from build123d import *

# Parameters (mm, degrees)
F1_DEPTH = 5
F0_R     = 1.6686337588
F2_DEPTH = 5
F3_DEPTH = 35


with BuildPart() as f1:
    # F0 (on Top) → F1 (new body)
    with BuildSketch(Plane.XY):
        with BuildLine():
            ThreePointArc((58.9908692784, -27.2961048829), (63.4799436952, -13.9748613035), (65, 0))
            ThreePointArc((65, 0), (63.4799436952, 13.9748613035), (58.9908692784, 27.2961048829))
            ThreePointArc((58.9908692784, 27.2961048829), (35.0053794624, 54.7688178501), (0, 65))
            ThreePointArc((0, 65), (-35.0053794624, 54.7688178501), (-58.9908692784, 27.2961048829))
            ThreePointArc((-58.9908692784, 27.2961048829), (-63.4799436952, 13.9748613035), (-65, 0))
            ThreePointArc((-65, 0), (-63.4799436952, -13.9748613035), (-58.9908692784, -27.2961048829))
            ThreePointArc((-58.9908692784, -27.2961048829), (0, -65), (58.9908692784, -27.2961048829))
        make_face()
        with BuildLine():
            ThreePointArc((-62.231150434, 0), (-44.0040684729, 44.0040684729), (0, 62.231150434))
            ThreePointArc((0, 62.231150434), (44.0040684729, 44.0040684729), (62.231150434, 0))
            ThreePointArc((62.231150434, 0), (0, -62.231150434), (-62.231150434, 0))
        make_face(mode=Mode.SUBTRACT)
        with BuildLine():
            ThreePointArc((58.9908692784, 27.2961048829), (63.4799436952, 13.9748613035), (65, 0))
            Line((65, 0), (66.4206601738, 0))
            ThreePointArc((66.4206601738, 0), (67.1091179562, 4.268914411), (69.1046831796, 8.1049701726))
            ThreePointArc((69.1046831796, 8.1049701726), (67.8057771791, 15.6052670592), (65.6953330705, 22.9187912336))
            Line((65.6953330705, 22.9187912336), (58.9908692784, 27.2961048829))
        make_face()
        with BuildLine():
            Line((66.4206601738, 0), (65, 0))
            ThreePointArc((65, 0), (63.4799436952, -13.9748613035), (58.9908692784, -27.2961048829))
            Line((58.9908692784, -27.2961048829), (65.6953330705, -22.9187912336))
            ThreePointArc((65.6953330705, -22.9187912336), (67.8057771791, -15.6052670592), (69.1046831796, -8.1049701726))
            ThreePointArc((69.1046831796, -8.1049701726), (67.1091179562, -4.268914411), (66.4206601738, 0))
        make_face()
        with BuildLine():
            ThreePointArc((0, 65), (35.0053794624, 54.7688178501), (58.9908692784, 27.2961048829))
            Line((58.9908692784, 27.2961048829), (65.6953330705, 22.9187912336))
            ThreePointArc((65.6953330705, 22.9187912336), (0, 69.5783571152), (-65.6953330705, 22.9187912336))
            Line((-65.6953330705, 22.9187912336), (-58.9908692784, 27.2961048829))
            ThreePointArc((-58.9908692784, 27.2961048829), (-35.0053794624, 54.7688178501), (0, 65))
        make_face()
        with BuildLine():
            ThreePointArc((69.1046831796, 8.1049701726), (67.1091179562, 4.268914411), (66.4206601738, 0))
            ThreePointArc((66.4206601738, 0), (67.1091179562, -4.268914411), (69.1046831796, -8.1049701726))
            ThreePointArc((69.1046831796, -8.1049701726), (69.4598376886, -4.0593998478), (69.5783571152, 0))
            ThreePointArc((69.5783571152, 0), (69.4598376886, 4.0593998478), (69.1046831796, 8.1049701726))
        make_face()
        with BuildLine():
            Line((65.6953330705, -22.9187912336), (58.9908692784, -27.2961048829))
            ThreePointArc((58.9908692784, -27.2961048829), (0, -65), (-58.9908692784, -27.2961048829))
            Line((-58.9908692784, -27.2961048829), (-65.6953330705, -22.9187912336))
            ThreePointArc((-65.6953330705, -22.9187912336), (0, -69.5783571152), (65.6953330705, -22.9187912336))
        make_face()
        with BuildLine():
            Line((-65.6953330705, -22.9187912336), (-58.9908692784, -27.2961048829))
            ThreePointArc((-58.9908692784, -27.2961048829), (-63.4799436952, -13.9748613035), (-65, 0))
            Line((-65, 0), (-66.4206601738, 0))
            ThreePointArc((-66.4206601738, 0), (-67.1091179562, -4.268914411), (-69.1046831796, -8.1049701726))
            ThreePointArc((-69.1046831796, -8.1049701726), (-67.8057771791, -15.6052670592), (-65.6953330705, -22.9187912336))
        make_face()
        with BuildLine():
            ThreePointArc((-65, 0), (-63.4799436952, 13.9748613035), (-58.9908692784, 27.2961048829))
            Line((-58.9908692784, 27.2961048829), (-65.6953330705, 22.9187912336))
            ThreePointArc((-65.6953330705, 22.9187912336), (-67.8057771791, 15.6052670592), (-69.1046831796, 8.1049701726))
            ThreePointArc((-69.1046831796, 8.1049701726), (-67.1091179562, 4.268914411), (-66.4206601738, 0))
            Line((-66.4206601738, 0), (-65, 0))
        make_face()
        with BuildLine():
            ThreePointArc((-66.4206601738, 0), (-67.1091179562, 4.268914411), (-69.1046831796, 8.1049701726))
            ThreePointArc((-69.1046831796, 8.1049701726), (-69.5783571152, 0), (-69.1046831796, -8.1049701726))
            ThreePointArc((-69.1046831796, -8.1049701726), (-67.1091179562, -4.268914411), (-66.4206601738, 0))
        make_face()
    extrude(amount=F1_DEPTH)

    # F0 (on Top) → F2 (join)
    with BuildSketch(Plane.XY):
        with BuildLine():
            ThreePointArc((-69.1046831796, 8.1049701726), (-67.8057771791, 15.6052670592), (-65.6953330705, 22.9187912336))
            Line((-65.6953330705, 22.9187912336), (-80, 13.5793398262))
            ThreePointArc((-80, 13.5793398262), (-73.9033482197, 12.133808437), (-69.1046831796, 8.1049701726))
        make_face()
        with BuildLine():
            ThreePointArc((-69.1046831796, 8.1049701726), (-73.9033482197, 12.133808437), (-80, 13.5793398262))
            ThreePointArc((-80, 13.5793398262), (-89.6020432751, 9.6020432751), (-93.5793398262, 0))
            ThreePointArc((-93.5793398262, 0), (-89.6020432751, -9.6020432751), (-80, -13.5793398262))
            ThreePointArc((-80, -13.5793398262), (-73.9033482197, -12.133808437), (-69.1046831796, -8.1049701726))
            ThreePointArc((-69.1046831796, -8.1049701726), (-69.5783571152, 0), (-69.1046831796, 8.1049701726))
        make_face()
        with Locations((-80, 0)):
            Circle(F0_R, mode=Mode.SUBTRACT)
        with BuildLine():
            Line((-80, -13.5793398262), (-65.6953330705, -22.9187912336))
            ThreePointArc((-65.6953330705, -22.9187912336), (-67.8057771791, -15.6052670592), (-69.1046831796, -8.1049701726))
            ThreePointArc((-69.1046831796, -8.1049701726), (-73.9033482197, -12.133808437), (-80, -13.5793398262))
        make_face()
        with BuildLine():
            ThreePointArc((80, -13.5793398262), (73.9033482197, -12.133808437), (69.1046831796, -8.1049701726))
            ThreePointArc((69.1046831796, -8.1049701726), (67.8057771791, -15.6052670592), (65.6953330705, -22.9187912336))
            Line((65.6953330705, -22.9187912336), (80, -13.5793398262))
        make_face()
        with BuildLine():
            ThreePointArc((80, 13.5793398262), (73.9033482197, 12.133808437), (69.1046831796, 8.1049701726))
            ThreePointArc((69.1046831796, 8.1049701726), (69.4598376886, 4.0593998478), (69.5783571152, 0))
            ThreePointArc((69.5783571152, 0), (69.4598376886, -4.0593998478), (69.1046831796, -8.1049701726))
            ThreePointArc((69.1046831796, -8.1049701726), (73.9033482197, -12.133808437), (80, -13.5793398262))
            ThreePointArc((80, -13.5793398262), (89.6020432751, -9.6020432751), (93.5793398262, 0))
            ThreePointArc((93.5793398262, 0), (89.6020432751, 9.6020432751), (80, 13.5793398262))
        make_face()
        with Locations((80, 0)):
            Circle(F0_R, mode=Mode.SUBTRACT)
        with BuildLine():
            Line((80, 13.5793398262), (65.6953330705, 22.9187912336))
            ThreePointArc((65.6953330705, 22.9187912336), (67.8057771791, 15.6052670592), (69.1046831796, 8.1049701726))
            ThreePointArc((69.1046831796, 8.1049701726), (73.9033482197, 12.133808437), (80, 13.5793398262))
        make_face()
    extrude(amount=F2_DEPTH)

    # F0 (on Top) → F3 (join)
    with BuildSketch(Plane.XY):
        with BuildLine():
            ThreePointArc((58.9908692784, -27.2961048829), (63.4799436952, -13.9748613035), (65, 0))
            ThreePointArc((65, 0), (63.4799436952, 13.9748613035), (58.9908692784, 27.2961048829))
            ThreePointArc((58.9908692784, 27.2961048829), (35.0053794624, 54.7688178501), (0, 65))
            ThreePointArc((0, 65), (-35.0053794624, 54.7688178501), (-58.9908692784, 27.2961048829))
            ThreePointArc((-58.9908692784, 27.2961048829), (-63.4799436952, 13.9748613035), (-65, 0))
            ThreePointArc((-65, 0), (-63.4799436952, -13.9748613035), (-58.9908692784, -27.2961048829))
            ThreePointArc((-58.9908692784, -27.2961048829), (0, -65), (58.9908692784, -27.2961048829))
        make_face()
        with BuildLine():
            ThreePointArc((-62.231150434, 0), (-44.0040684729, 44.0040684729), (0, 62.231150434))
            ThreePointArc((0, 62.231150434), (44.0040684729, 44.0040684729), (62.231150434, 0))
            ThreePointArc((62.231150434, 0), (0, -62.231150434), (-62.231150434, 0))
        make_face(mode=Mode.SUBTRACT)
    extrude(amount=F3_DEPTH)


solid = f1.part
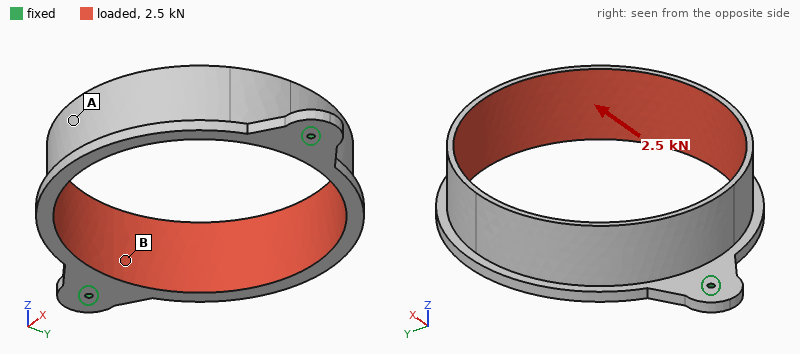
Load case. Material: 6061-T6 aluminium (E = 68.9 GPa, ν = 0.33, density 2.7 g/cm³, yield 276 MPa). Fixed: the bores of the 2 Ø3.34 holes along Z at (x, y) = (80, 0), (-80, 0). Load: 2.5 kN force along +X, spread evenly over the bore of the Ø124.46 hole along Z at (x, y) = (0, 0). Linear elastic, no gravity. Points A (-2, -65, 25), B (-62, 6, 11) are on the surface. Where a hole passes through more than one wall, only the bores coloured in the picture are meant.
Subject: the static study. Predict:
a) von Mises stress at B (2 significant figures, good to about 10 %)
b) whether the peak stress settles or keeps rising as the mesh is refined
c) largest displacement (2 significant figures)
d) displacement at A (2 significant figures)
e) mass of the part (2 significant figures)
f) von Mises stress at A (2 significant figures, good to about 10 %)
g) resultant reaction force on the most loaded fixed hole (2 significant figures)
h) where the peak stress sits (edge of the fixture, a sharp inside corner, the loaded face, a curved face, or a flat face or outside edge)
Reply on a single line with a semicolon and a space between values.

20 MPa; keeps rising; 0.16 mm; 0.12 mm; 150 g; 7.4 MPa; 1.3 kN; a sharp inside corner
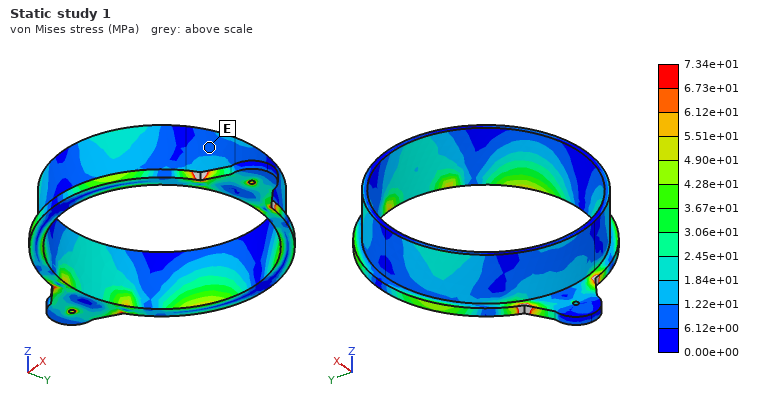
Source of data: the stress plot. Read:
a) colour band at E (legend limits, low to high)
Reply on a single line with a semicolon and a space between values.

6.12e+00 to 1.22e+01 MPa
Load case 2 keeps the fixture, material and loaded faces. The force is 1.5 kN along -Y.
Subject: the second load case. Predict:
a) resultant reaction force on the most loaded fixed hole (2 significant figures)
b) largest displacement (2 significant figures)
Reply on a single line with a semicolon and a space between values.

750 N; 0.64 mm
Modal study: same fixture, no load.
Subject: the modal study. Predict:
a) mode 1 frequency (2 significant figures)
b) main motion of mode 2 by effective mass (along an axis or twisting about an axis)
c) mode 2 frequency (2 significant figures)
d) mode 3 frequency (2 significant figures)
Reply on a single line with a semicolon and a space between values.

480 Hz; along Z; 760 Hz; 1100 Hz
